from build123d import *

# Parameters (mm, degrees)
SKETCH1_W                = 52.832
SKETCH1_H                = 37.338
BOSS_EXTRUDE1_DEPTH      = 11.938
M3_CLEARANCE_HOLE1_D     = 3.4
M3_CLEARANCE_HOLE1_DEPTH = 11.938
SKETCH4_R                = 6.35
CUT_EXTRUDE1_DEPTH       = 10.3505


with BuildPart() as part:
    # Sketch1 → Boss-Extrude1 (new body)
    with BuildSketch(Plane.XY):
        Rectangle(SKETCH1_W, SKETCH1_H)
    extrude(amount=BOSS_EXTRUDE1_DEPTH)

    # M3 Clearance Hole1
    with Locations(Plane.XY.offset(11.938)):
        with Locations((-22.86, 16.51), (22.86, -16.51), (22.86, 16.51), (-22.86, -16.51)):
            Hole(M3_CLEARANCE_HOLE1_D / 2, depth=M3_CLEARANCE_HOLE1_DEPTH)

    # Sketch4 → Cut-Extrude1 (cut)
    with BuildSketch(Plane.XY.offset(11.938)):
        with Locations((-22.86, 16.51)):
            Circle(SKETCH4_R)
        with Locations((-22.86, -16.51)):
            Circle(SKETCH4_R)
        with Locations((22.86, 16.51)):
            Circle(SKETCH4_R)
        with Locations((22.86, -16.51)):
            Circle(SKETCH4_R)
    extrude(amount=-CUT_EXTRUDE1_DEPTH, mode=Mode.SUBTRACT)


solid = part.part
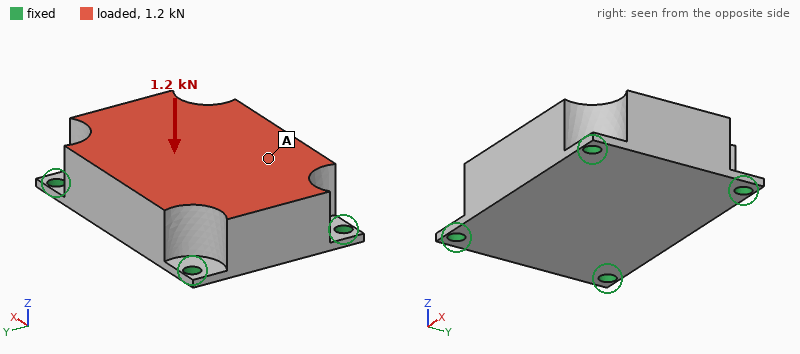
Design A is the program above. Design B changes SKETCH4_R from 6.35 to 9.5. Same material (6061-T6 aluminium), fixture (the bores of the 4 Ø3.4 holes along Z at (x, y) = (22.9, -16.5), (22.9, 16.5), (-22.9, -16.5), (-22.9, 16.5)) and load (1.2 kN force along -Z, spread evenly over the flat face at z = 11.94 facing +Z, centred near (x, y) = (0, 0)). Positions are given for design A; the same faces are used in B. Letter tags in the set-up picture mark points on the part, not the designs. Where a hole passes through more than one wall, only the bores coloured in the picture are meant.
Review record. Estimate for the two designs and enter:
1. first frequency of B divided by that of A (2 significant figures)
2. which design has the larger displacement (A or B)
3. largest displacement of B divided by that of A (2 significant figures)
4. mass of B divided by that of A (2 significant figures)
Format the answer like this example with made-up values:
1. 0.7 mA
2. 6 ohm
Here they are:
1. 0.66
2. B
3. 2.6
4. 0.88
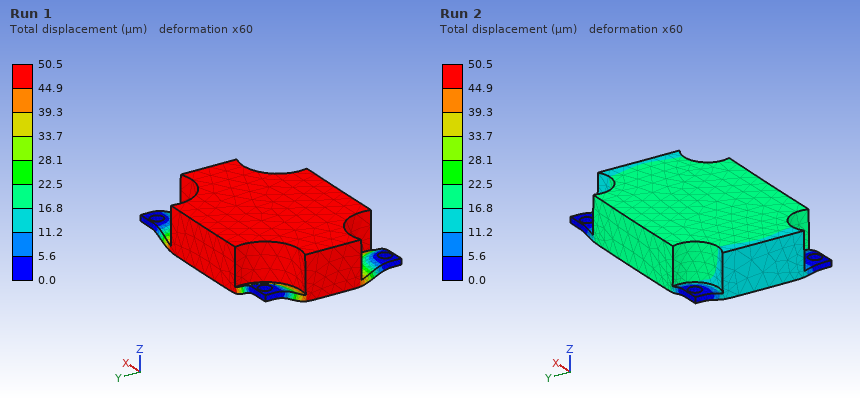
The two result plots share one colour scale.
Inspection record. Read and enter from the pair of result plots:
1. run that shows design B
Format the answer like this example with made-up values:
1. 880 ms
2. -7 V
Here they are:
1. Run 1
